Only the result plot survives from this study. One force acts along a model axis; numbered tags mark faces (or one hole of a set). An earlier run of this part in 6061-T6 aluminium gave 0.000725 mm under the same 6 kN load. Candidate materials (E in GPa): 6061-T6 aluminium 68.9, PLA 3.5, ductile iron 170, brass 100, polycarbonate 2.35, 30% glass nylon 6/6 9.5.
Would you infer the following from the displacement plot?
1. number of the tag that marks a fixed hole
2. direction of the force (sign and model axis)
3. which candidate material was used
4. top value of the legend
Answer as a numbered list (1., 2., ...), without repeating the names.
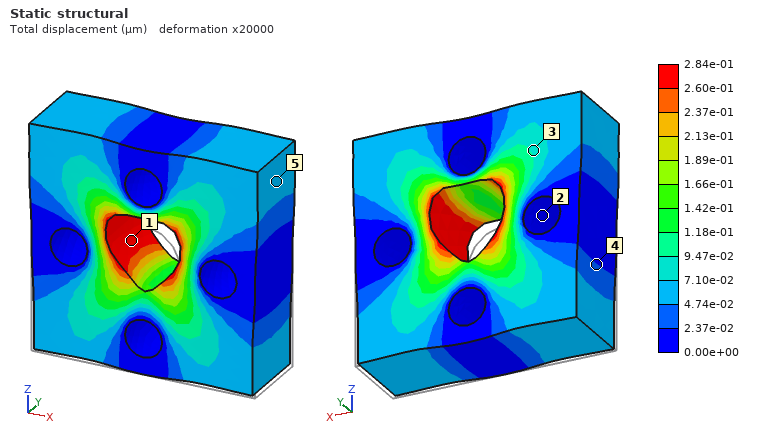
1. 2
2. +Z
3. ductile iron
4. 2.84e-01 µm
